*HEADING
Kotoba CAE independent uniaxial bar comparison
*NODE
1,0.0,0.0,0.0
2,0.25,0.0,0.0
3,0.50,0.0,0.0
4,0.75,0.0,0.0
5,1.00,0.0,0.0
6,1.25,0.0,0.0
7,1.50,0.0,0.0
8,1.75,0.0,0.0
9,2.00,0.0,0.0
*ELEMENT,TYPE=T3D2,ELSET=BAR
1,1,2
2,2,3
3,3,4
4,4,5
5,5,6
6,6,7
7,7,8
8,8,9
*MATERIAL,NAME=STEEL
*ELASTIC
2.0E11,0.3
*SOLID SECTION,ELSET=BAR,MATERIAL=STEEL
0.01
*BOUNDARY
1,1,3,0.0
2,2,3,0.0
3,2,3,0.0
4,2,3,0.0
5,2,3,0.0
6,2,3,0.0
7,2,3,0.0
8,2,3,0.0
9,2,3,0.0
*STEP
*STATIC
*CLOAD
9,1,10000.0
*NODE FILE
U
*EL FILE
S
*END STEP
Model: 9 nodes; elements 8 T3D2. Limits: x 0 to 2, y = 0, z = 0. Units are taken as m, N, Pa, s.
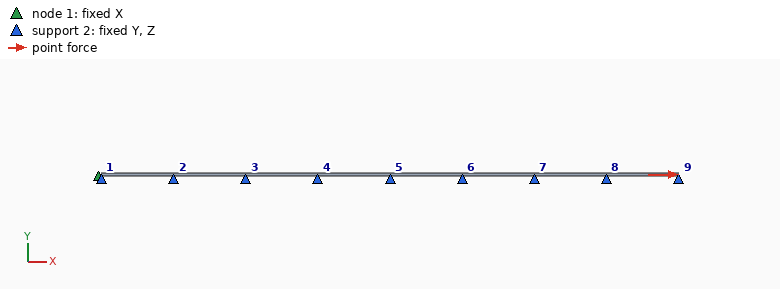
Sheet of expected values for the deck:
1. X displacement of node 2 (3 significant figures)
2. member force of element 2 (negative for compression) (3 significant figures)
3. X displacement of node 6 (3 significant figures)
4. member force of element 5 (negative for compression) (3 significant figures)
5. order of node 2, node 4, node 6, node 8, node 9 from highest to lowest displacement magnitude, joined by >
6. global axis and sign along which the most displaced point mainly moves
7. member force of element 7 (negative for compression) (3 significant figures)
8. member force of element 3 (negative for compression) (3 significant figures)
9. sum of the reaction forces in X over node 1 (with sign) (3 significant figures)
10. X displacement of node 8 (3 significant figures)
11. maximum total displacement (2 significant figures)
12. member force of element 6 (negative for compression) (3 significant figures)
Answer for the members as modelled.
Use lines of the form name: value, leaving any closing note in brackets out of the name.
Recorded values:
X displacement of node 2: 1.25e-06 m
member force of element 2 (negative for compression): 10000 N
X displacement of node 6: 6.25e-06 m
member force of element 5 (negative for compression): 10000 N
order of node 2, node 4, node 6, node 8, node 9 from highest to lowest displacement magnitude, joined by >: node 9 > node 8 > node 6 > node 4 > node 2
global axis and sign along which the most displaced point mainly moves: +X
member force of element 7 (negative for compression): 10000 N
member force of element 3 (negative for compression): 10000 N
sum of the reaction forces in X over node 1 (with sign): -10000 N
X displacement of node 8: 8.75e-06 m
maximum total displacement: 1.0e-05 m
member force of element 6 (negative for compression): 10000 N
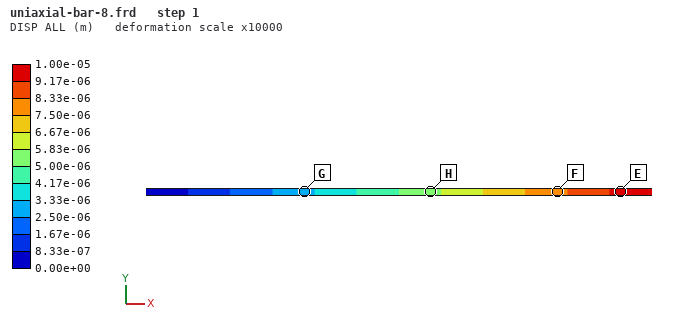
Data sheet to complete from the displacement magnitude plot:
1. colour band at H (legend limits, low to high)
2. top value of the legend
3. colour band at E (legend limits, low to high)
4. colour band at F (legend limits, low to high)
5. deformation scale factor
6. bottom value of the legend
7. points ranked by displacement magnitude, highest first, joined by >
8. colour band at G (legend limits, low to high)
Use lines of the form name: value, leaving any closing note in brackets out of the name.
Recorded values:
colour band at H: 5.00e-06 to 5.83e-06 m
top value of the legend: 1.00e-05 m
colour band at E: 9.17e-06 to 1.00e-05 m
colour band at F: 7.50e-06 to 8.33e-06 m
deformation scale factor: 10000
bottom value of the legend: 0.00e+00 m
points ranked by displacement magnitude, highest first, joined by >: E > F > H > G
colour band at G: 2.50e-06 to 3.33e-06 m
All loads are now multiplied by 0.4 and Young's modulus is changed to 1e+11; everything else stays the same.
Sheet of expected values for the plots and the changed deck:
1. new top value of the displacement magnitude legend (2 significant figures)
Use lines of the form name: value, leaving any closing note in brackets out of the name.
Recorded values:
new top value of the displacement magnitude legend: 8.0e-06 m
